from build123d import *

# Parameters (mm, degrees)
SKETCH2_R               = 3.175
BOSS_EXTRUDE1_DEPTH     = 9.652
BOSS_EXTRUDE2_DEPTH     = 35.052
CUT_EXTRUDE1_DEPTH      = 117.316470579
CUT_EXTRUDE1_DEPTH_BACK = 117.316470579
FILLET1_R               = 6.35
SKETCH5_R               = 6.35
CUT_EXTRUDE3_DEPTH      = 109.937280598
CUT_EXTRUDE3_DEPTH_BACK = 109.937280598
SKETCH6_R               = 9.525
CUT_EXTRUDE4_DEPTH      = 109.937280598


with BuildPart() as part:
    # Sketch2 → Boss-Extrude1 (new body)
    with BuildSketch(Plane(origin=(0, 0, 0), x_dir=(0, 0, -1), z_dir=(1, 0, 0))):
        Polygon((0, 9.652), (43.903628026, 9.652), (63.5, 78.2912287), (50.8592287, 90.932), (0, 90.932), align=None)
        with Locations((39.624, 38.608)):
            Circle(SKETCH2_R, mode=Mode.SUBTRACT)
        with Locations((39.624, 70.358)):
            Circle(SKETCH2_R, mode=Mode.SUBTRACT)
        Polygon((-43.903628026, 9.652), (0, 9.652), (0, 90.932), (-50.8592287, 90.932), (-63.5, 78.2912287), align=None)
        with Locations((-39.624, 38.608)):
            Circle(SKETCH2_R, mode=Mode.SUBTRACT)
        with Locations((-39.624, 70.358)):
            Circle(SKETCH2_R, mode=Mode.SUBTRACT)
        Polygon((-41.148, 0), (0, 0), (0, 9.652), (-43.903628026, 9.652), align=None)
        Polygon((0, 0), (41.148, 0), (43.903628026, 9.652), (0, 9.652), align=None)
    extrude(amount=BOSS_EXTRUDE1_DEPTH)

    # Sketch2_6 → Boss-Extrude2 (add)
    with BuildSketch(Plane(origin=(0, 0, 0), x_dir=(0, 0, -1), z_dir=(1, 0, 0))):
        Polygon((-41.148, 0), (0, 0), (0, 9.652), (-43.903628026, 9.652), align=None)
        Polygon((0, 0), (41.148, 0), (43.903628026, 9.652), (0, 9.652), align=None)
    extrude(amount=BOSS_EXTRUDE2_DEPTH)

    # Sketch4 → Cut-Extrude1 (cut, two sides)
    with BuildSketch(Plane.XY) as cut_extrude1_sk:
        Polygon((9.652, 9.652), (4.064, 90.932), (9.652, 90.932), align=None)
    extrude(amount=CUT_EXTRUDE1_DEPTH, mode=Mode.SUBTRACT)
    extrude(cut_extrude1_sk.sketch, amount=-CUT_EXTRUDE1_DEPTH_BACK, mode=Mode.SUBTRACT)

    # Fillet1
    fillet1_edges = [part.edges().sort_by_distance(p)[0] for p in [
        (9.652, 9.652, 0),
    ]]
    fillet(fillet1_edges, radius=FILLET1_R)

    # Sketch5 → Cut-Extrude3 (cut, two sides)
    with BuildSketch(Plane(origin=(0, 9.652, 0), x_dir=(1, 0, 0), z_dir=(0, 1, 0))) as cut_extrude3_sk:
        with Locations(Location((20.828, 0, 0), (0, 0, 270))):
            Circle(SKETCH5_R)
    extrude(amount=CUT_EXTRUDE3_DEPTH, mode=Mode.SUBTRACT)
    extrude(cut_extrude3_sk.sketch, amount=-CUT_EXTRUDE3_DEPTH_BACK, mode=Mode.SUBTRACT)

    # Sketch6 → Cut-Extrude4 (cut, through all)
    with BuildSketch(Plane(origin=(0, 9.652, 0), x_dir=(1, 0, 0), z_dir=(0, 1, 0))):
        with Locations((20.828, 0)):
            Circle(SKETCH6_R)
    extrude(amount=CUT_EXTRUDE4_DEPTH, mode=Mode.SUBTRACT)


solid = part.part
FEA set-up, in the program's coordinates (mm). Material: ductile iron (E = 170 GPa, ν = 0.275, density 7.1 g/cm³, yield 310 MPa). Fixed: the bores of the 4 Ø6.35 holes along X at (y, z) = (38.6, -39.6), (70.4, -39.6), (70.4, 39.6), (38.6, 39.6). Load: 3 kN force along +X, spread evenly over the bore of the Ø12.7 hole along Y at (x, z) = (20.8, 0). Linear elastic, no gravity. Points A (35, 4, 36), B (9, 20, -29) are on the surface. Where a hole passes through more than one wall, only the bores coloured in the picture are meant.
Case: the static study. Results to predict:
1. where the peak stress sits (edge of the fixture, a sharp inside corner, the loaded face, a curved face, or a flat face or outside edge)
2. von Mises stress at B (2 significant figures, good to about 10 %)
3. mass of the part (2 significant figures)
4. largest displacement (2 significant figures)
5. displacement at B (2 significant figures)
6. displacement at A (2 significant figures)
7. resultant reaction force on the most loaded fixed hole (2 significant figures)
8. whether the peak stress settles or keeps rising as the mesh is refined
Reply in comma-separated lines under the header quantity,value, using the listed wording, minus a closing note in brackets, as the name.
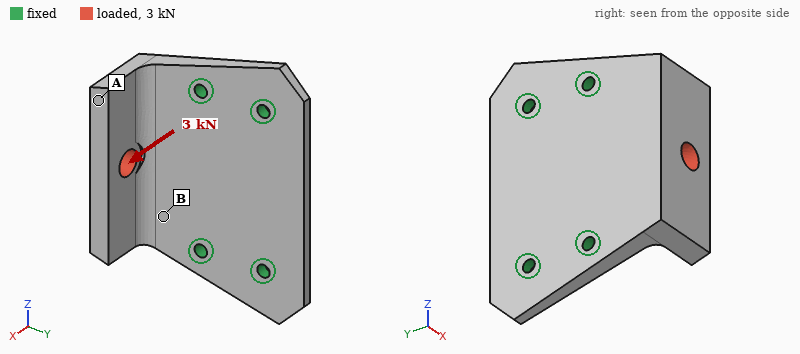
quantity,value
where the peak stress sits,edge of the fixture
von Mises stress at B,35 MPa
mass of the part,610 g
largest displacement,0.12 mm
displacement at B,0.037 mm
displacement at A,0.11 mm
resultant reaction force on the most loaded fixed hole,2.0 kN
whether the peak stress settles or keeps rising as the mesh is refined,keeps rising
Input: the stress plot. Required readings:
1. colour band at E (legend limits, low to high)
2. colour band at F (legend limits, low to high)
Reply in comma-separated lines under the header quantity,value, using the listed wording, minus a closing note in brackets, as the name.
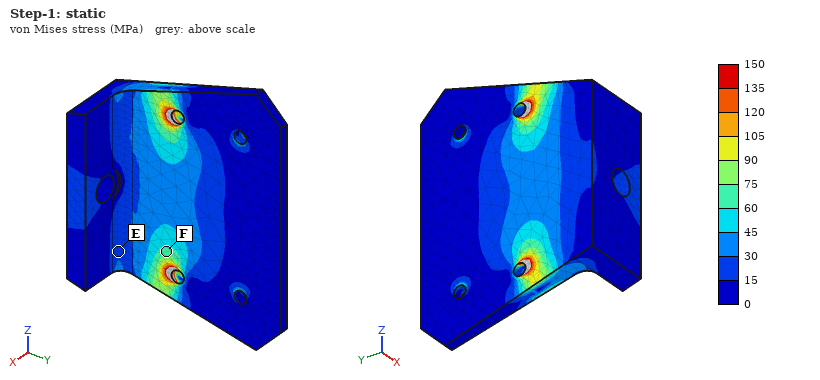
quantity,value
colour band at E,15 to 30 MPa
colour band at F,60 to 75 MPa
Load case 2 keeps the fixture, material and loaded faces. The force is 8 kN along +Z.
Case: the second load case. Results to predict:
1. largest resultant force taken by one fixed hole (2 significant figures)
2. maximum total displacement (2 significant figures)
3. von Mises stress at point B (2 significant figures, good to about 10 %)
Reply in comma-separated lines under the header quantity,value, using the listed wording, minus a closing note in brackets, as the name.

quantity,value
largest resultant force taken by one fixed hole,5.0 kN
maximum total displacement,54 µm
von Mises stress at point B,55 MPa
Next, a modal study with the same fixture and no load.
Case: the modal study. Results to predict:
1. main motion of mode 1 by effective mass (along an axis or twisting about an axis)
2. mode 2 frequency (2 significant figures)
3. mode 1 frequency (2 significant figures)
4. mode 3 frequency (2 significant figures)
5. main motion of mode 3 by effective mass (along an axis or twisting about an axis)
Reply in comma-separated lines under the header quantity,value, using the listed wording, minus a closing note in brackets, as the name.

quantity,value
main motion of mode 1 by effective mass,along X
mode 2 frequency,4000 Hz
mode 1 frequency,1800 Hz
mode 3 frequency,4400 Hz
main motion of mode 3 by effective mass,along X
